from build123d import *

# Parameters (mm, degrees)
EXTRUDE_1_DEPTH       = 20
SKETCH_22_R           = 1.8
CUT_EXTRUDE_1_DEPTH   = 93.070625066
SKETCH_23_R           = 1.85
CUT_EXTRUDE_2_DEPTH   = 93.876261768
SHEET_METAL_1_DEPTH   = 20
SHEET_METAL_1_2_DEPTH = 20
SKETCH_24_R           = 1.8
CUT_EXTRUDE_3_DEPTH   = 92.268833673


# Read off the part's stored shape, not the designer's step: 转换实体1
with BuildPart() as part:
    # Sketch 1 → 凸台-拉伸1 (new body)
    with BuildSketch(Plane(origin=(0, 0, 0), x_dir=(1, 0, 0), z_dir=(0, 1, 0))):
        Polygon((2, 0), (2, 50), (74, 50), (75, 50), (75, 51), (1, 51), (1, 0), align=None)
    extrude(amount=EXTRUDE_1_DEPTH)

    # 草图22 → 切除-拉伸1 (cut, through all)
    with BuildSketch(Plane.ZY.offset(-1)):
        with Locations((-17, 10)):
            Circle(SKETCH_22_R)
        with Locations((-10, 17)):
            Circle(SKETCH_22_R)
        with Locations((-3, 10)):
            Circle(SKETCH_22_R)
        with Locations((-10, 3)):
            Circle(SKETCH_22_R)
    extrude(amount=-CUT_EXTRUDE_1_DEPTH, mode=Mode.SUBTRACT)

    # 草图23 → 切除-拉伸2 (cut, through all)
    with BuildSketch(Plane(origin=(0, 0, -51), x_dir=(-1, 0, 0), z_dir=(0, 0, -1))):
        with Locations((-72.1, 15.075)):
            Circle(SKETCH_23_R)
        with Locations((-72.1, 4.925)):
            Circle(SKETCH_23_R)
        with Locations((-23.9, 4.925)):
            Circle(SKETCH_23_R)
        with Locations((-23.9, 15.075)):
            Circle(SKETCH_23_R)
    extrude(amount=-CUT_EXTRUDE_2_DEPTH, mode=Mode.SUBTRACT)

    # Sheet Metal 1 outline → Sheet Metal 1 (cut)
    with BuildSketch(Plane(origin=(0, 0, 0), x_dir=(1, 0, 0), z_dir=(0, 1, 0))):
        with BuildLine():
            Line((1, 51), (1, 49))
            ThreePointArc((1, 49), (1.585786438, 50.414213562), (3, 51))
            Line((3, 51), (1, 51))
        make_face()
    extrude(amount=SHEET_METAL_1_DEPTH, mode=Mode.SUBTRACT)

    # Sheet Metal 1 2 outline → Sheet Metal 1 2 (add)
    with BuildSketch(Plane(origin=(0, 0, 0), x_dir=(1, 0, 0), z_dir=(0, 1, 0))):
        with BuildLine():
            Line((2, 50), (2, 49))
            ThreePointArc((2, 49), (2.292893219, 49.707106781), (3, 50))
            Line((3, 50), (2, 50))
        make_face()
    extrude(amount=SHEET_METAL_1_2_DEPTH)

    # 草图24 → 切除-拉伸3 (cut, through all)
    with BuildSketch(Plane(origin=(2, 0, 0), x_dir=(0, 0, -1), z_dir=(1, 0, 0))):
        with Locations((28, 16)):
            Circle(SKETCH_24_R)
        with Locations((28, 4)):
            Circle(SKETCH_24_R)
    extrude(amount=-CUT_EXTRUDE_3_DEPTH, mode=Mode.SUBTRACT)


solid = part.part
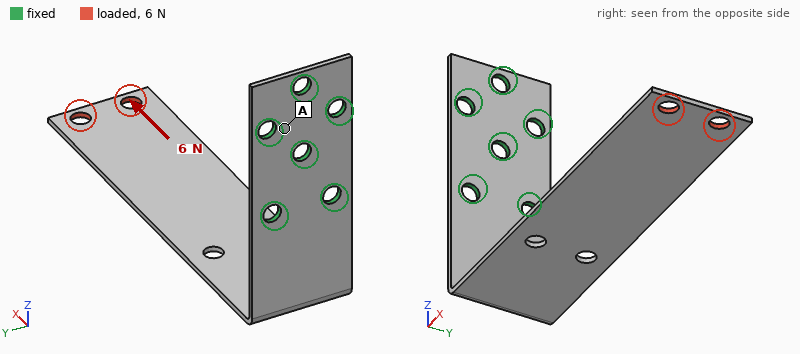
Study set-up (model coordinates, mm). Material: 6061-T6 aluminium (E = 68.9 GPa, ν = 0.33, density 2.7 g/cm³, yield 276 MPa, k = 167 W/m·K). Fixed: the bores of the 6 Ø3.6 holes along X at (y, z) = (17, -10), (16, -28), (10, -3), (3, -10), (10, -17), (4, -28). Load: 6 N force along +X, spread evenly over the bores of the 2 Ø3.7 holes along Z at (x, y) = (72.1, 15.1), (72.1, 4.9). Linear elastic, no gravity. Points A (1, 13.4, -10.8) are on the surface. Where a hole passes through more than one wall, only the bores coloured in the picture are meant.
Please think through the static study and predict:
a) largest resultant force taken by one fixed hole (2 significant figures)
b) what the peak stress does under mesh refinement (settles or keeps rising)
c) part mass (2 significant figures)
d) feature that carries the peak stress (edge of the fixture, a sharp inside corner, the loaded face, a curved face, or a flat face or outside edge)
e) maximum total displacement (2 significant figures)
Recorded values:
3.3 N
keeps rising
6.4 g
edge of the fixture
0.84 mm
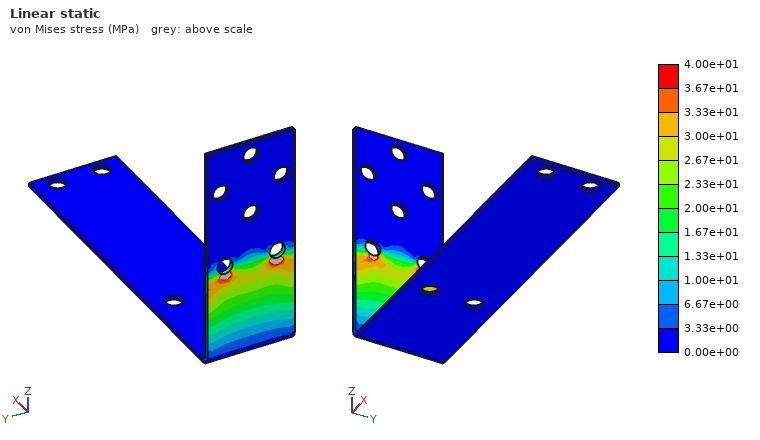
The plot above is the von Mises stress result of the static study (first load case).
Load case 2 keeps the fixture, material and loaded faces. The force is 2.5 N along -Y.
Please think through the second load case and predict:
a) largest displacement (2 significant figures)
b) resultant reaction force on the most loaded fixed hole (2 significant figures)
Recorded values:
1.1 mm
13 N
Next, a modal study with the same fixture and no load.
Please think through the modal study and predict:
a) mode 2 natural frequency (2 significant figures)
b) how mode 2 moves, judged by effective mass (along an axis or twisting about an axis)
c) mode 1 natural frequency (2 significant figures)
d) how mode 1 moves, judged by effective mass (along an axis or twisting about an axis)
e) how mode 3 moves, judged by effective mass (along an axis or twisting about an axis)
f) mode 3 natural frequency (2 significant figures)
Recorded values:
210 Hz
along Y
110 Hz
along Z
along X
560 Hz
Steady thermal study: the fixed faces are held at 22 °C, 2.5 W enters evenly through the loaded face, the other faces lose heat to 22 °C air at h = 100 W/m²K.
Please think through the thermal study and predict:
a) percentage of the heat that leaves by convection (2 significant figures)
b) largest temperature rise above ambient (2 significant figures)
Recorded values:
93 %
21 K
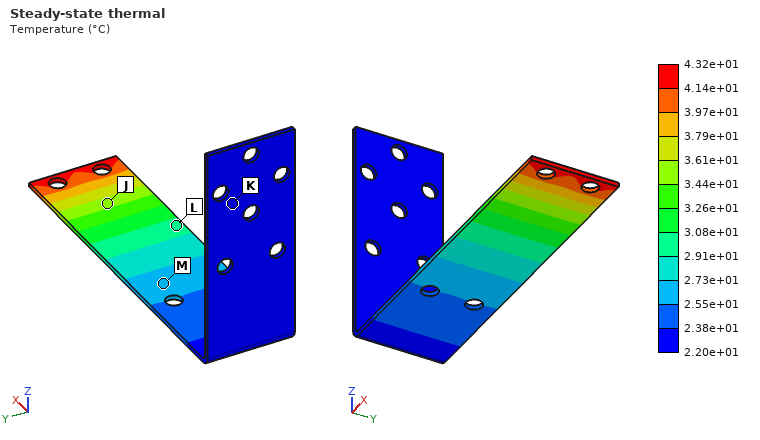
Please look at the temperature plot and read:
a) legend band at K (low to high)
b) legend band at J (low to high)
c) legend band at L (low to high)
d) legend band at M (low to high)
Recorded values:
2.20e+01 to 2.38e+01 °C
3.44e+01 to 3.61e+01 °C
2.91e+01 to 3.08e+01 °C
2.55e+01 to 2.73e+01 °C
